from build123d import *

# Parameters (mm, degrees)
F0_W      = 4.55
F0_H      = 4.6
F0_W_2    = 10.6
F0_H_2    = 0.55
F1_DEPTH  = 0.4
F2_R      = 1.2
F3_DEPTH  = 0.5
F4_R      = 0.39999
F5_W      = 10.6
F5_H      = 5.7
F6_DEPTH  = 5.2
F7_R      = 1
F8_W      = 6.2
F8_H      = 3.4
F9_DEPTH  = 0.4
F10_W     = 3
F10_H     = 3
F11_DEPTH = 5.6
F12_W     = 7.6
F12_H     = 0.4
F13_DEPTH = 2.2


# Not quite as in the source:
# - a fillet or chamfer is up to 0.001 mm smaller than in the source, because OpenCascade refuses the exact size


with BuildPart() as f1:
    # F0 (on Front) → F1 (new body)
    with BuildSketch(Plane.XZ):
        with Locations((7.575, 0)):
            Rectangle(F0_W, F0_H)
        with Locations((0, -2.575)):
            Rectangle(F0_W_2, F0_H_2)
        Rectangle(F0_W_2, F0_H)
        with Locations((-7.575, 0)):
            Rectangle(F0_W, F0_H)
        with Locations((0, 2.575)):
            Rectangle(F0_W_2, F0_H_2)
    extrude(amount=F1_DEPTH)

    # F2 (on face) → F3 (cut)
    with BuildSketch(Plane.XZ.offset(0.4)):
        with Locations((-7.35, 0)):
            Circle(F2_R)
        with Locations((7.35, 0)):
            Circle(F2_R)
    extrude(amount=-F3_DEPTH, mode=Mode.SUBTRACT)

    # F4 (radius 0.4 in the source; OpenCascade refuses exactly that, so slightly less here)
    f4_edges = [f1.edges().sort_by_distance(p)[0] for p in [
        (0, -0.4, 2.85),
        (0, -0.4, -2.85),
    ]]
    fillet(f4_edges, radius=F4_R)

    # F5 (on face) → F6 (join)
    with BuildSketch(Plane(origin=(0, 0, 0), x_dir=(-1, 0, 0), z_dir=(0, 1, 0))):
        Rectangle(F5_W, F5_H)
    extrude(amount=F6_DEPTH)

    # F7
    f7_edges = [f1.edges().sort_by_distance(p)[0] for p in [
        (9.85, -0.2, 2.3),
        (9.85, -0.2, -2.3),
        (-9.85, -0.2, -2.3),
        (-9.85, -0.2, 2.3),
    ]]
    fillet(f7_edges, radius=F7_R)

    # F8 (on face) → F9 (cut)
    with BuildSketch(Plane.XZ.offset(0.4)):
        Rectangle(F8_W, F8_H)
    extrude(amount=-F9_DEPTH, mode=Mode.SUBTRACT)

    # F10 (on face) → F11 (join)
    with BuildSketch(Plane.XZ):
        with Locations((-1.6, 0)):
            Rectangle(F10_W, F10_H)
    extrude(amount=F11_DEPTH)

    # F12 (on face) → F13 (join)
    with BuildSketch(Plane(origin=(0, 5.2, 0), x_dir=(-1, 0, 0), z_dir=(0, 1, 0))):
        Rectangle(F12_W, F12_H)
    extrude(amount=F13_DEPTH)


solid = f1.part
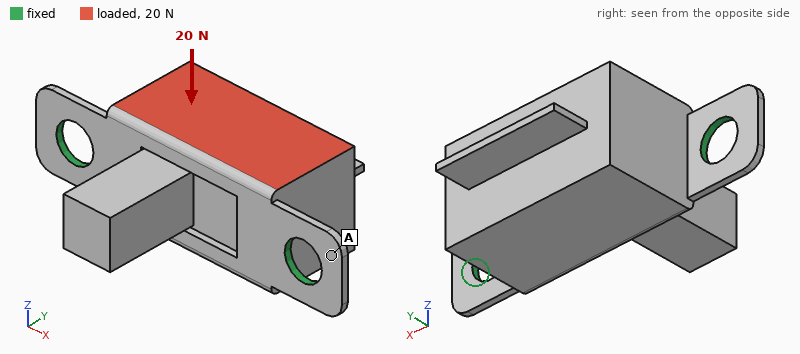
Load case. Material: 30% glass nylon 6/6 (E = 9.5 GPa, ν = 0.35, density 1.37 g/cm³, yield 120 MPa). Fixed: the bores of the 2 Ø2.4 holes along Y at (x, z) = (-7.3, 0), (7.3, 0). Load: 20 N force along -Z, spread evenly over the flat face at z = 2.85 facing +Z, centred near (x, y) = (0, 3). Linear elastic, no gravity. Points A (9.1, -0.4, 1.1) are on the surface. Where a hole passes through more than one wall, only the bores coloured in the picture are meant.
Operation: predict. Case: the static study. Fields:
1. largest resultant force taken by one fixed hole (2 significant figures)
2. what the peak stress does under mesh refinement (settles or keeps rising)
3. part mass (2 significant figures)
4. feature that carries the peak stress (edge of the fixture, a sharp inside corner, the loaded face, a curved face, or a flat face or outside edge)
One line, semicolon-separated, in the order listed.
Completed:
10 N; keeps rising; 0.55 g; edge of the fixture
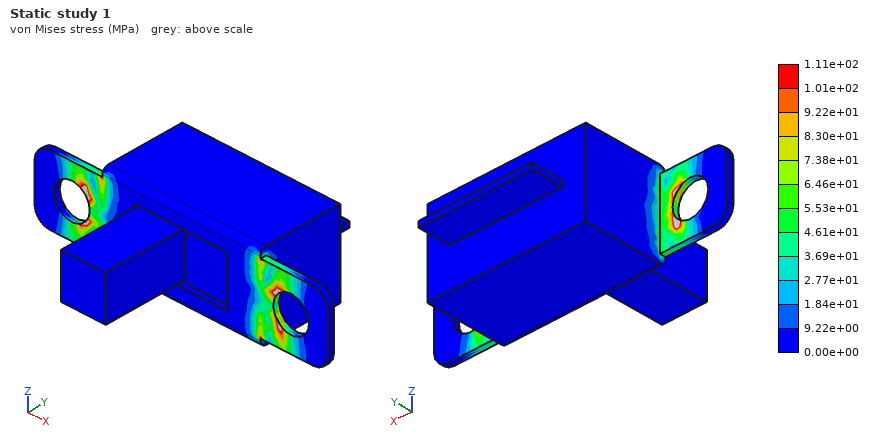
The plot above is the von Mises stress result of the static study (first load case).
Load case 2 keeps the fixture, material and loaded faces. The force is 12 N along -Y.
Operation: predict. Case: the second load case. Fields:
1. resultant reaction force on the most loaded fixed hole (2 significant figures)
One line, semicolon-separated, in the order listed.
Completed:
7.2 N
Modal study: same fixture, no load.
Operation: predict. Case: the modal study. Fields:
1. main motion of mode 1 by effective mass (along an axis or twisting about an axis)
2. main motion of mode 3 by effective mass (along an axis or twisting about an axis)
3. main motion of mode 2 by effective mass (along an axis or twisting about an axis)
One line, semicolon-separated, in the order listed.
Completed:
along Z; along X; along Y
